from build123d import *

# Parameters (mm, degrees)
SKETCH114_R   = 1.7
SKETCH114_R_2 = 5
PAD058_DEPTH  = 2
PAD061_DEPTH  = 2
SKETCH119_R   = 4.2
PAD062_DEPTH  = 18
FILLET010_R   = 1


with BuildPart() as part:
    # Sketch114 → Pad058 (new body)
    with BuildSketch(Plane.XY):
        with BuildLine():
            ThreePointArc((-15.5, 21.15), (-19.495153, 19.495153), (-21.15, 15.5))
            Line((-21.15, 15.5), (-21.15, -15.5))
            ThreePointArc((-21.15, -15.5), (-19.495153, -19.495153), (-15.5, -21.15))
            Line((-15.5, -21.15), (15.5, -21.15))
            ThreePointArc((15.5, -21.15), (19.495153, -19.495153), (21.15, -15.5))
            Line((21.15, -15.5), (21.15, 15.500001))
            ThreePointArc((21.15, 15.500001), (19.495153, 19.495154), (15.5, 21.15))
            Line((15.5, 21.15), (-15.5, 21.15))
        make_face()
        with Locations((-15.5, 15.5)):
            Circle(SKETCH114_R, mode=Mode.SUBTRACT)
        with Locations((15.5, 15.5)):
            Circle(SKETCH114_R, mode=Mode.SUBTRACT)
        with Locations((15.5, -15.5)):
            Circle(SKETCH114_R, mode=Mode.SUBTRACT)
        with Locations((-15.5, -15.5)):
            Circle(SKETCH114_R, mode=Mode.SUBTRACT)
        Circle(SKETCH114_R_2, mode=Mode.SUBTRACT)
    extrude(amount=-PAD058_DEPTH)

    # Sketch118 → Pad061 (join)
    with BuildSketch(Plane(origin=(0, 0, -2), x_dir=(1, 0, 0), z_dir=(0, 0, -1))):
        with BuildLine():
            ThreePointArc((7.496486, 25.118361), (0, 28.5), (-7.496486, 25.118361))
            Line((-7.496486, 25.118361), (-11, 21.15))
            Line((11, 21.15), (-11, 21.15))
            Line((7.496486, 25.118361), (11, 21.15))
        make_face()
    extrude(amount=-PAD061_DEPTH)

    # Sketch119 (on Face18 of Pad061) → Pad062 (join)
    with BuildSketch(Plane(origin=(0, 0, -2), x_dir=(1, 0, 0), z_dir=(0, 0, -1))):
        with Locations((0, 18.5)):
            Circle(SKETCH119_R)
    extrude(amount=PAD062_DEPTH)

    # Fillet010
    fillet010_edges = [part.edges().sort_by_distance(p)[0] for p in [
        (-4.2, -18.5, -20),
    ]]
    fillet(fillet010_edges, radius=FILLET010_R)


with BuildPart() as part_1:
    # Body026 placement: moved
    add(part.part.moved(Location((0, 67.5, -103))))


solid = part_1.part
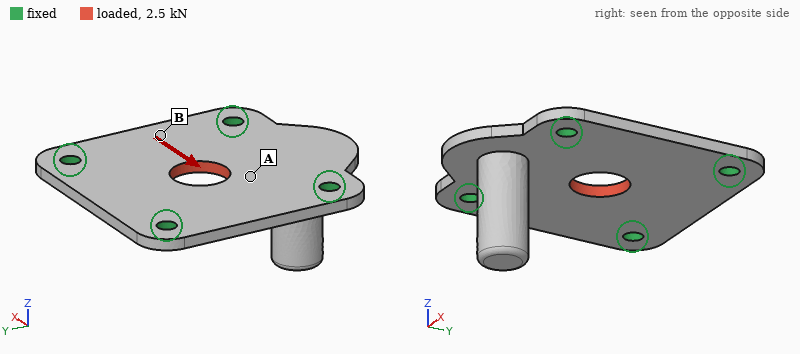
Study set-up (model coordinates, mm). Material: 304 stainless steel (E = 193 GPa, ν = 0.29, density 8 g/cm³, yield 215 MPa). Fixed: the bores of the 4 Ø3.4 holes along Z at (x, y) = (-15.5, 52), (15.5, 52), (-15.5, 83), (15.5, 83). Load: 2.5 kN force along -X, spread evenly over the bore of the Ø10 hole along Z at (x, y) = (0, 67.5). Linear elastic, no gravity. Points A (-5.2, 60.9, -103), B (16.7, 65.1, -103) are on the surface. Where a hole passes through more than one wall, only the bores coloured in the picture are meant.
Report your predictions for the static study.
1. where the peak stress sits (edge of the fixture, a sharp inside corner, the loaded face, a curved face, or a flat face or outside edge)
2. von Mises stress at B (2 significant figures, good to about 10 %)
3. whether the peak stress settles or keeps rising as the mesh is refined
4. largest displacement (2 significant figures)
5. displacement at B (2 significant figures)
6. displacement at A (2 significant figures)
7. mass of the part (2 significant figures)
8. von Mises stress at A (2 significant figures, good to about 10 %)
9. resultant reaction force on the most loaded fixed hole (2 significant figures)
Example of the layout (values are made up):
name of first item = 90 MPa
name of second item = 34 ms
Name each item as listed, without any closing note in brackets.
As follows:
where the peak stress sits = edge of the fixture
von Mises stress at B = 12 MPa
whether the peak stress settles or keeps rising as the mesh is refined = keeps rising
largest displacement = 4.1 µm
displacement at B = 2.7 µm
displacement at A = 2.7 µm
mass of the part = 36 g
von Mises stress at A = 34 MPa
resultant reaction force on the most loaded fixed hole = 680 N
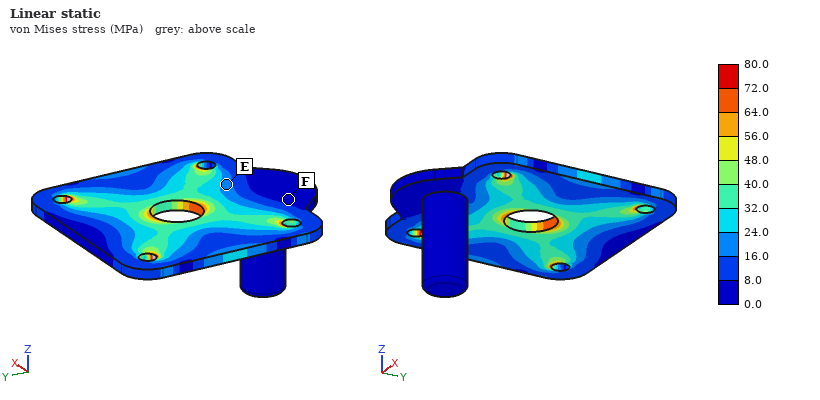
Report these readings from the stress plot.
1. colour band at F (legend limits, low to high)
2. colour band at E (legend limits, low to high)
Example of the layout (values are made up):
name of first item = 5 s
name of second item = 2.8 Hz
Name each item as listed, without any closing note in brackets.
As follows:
colour band at F = 0.0 to 8.0 MPa
colour band at E = 16.0 to 24.0 MPa
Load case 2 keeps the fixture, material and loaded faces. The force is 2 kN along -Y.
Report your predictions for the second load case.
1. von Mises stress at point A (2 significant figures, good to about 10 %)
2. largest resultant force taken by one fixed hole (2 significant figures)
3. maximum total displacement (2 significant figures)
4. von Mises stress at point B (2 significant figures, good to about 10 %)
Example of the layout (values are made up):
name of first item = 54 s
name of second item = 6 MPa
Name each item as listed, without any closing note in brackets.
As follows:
von Mises stress at point A = 26 MPa
largest resultant force taken by one fixed hole = 540 N
maximum total displacement = 3.2 µm
von Mises stress at point B = 6.8 MPa
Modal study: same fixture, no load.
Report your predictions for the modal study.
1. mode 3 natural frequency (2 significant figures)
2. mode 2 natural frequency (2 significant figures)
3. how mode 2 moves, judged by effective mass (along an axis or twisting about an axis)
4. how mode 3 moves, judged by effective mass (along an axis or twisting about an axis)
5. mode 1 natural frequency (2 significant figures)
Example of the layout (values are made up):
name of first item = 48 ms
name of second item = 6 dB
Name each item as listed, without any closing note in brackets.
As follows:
mode 3 natural frequency = 6600 Hz
mode 2 natural frequency = 6200 Hz
how mode 2 moves, judged by effective mass = along X
how mode 3 moves, judged by effective mass = along Z
mode 1 natural frequency = 3500 Hz
